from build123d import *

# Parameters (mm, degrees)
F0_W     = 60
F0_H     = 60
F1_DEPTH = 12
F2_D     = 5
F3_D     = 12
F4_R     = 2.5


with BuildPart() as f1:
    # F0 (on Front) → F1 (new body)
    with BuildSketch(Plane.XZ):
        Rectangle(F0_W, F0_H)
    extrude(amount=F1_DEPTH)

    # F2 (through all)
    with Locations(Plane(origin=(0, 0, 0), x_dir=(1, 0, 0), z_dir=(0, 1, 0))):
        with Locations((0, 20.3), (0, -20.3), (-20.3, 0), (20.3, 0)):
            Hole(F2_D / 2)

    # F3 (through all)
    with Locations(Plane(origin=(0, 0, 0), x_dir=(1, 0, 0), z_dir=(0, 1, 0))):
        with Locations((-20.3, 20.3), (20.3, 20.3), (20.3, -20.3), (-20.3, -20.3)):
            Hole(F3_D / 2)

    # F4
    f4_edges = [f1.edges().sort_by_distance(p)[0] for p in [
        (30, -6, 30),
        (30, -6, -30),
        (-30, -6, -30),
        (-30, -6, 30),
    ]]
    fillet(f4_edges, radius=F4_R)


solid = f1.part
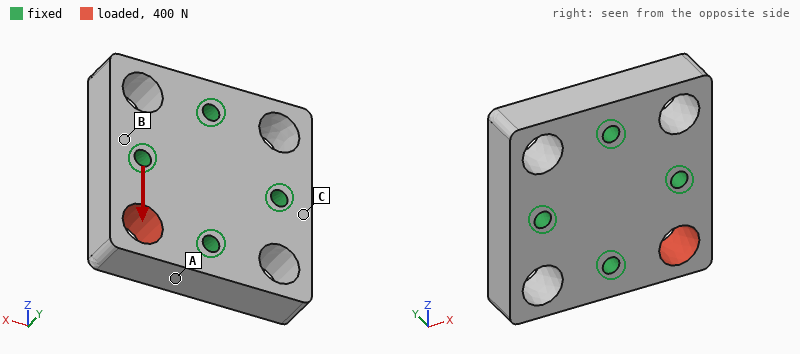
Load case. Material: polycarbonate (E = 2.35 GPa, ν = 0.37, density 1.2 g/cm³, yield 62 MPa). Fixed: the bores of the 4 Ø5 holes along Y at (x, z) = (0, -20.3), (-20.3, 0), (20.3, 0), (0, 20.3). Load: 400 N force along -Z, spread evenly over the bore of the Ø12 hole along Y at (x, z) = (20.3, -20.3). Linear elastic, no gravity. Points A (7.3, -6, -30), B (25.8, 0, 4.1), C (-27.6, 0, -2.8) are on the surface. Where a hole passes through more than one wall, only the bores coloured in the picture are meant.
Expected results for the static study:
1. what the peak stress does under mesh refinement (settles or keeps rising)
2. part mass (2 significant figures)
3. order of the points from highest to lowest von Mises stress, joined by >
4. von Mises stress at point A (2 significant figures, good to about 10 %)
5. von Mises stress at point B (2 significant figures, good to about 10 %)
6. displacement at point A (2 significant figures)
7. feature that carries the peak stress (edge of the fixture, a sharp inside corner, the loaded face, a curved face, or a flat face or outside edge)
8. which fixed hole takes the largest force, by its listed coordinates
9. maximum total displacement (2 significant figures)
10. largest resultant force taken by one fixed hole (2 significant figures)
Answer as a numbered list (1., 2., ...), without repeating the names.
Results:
1. keeps rising
2. 44 g
3. A > B > C
4. 1.5 MPa
5. 0.77 MPa
6. 10 µm
7. a sharp inside corner
8. (20.3, 0)
9. 37 µm
10. 290 N
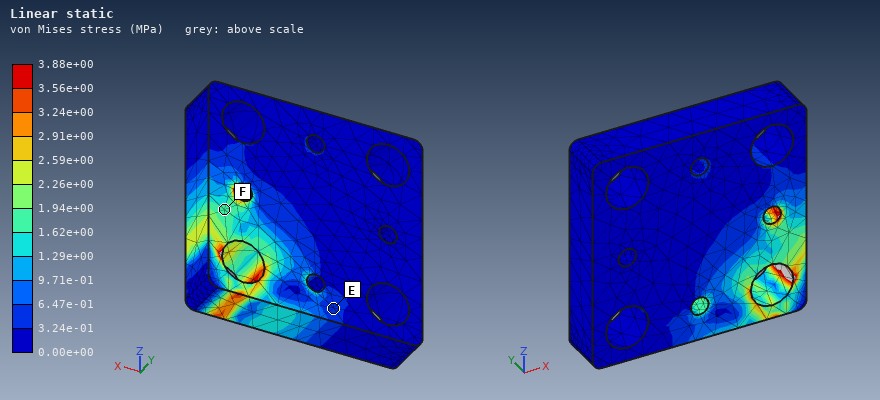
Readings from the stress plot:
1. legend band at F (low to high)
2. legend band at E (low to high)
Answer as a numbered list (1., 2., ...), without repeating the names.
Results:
1. 1.62e+00 to 1.94e+00 MPa
2. 3.24e-01 to 6.47e-01 MPa
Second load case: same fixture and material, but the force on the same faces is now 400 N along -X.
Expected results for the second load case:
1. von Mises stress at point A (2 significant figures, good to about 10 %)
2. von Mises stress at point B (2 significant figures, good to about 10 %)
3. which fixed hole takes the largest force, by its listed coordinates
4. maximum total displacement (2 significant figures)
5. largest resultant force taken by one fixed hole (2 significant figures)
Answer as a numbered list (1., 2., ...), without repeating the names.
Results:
1. 2.0 MPa
2. 0.54 MPa
3. (0, -20.3)
4. 37 µm
5. 290 N
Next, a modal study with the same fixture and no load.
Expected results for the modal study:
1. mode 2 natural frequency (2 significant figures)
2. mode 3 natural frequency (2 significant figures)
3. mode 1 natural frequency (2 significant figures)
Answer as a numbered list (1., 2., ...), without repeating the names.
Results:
1. 4800 Hz
2. 4800 Hz
3. 4600 Hz
